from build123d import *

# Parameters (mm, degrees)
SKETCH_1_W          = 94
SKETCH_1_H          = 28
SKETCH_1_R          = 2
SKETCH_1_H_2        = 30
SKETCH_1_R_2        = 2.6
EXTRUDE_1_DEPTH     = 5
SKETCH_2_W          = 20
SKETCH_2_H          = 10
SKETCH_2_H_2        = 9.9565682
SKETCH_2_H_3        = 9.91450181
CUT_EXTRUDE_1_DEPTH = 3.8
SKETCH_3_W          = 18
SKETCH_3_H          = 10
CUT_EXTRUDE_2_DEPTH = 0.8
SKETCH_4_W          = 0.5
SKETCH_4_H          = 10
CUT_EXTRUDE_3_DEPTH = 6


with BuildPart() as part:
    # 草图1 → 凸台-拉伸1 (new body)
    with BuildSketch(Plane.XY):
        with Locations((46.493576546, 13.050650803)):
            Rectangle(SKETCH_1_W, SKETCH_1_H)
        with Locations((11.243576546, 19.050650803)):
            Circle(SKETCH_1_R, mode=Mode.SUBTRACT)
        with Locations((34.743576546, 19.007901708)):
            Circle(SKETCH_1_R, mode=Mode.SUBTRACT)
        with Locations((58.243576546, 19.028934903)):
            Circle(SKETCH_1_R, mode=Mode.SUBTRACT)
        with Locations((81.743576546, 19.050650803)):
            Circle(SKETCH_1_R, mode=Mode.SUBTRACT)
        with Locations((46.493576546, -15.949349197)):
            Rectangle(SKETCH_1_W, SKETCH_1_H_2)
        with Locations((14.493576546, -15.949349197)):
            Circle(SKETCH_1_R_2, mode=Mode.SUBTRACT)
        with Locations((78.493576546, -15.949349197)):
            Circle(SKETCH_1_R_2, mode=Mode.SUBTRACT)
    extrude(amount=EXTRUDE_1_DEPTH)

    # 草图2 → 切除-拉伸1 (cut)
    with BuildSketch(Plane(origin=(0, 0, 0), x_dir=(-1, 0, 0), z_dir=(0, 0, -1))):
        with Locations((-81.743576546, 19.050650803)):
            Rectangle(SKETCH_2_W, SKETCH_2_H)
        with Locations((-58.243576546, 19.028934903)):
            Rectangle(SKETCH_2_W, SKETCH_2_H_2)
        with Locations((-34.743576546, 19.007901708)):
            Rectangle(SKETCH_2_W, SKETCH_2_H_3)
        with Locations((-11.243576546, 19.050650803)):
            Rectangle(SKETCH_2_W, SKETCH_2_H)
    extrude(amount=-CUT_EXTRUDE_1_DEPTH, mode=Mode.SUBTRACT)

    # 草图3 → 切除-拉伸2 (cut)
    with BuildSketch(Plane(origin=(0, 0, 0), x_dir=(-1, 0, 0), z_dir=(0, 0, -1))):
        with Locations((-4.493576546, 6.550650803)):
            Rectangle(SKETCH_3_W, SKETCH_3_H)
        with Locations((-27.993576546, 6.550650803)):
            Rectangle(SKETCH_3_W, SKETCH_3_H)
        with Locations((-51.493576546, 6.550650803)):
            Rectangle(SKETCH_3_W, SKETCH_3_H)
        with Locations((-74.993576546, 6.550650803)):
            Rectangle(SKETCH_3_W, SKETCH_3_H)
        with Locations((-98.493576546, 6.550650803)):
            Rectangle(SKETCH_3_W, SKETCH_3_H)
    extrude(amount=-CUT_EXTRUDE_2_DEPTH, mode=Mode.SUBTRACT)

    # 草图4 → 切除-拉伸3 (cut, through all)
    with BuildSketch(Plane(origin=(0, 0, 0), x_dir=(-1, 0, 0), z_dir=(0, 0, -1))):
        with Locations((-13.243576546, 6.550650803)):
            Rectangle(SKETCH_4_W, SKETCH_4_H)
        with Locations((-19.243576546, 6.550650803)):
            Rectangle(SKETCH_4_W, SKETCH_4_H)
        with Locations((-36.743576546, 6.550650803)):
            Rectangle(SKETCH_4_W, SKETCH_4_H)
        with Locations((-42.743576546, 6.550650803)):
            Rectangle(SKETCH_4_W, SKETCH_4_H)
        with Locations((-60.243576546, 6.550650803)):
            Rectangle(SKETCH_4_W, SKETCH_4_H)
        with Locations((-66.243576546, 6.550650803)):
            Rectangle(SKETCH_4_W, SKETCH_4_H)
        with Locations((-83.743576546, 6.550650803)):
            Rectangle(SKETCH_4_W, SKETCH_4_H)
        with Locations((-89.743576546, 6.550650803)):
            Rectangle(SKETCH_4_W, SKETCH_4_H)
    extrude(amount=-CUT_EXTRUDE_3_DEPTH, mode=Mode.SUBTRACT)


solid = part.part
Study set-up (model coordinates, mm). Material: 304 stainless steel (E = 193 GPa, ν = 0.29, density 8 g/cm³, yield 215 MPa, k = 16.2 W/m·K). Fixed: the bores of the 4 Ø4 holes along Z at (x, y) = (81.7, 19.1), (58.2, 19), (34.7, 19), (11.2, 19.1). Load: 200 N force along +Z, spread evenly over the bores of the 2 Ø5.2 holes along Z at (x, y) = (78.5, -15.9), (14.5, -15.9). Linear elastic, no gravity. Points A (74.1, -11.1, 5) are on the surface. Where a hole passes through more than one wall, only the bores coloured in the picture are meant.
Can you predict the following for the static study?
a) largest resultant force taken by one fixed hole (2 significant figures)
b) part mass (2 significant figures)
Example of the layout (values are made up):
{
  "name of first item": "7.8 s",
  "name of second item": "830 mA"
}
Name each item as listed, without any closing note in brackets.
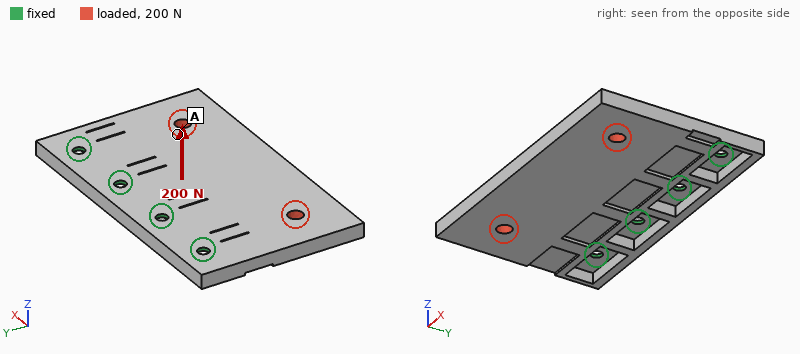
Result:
{
  "largest resultant force taken by one fixed hole": "70 N",
  "part mass": "190 g"
}
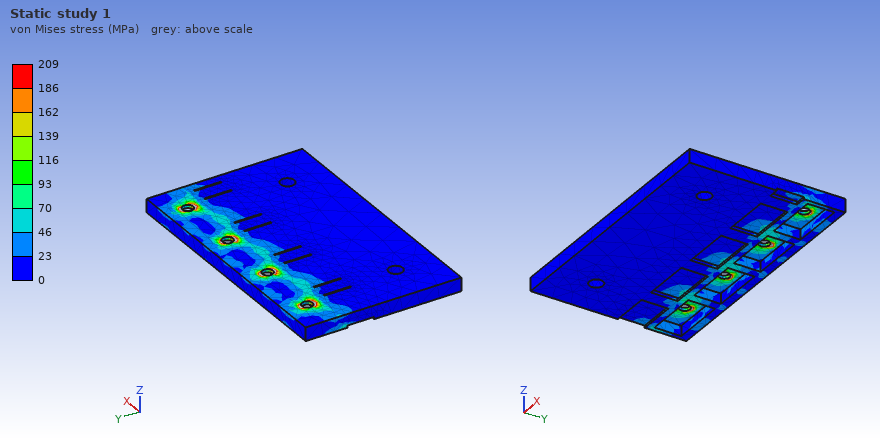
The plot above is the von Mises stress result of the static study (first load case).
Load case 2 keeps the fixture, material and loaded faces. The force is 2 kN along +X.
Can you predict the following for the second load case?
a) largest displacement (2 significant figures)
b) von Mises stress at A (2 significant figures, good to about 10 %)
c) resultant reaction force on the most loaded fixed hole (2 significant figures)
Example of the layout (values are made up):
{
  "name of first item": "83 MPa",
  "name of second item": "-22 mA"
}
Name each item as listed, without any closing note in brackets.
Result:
{
  "largest displacement": "20 µm",
  "von Mises stress at A": "15 MPa",
  "resultant reaction force on the most loaded fixed hole": "1000 N"
}
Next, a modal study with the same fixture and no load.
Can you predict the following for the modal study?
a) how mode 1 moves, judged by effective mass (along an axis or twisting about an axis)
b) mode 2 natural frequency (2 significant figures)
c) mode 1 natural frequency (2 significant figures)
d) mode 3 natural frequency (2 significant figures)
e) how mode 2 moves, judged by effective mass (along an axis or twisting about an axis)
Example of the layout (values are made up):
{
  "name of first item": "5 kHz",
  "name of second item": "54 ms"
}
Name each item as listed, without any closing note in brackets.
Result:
{
  "how mode 1 moves, judged by effective mass": "along Z",
  "mode 2 natural frequency": "1500 Hz",
  "mode 1 natural frequency": "540 Hz",
  "mode 3 natural frequency": "3800 Hz",
  "how mode 2 moves, judged by effective mass": "twisting about Y"
}
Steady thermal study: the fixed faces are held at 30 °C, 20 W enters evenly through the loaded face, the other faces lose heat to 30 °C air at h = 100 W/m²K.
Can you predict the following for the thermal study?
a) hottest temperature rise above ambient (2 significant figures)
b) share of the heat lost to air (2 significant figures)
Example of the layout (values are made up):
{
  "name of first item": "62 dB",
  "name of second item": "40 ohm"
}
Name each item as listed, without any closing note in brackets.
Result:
{
  "hottest temperature rise above ambient": "56 K",
  "share of the heat lost to air": "94 %"
}
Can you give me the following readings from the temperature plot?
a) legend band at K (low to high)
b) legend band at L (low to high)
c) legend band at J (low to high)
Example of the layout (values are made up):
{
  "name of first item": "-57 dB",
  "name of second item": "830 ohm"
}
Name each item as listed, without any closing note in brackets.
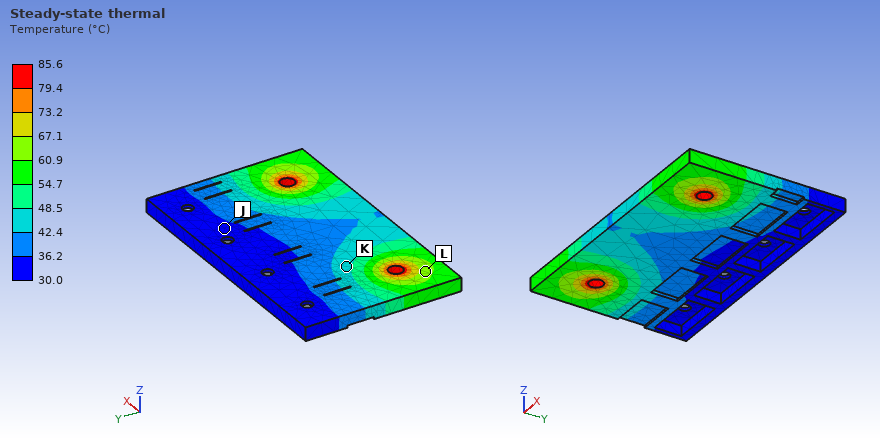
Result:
{
  "legend band at K": "42.4 to 48.5 °C",
  "legend band at L": "60.9 to 67.1 °C",
  "legend band at J": "30.0 to 36.2 °C"
}
